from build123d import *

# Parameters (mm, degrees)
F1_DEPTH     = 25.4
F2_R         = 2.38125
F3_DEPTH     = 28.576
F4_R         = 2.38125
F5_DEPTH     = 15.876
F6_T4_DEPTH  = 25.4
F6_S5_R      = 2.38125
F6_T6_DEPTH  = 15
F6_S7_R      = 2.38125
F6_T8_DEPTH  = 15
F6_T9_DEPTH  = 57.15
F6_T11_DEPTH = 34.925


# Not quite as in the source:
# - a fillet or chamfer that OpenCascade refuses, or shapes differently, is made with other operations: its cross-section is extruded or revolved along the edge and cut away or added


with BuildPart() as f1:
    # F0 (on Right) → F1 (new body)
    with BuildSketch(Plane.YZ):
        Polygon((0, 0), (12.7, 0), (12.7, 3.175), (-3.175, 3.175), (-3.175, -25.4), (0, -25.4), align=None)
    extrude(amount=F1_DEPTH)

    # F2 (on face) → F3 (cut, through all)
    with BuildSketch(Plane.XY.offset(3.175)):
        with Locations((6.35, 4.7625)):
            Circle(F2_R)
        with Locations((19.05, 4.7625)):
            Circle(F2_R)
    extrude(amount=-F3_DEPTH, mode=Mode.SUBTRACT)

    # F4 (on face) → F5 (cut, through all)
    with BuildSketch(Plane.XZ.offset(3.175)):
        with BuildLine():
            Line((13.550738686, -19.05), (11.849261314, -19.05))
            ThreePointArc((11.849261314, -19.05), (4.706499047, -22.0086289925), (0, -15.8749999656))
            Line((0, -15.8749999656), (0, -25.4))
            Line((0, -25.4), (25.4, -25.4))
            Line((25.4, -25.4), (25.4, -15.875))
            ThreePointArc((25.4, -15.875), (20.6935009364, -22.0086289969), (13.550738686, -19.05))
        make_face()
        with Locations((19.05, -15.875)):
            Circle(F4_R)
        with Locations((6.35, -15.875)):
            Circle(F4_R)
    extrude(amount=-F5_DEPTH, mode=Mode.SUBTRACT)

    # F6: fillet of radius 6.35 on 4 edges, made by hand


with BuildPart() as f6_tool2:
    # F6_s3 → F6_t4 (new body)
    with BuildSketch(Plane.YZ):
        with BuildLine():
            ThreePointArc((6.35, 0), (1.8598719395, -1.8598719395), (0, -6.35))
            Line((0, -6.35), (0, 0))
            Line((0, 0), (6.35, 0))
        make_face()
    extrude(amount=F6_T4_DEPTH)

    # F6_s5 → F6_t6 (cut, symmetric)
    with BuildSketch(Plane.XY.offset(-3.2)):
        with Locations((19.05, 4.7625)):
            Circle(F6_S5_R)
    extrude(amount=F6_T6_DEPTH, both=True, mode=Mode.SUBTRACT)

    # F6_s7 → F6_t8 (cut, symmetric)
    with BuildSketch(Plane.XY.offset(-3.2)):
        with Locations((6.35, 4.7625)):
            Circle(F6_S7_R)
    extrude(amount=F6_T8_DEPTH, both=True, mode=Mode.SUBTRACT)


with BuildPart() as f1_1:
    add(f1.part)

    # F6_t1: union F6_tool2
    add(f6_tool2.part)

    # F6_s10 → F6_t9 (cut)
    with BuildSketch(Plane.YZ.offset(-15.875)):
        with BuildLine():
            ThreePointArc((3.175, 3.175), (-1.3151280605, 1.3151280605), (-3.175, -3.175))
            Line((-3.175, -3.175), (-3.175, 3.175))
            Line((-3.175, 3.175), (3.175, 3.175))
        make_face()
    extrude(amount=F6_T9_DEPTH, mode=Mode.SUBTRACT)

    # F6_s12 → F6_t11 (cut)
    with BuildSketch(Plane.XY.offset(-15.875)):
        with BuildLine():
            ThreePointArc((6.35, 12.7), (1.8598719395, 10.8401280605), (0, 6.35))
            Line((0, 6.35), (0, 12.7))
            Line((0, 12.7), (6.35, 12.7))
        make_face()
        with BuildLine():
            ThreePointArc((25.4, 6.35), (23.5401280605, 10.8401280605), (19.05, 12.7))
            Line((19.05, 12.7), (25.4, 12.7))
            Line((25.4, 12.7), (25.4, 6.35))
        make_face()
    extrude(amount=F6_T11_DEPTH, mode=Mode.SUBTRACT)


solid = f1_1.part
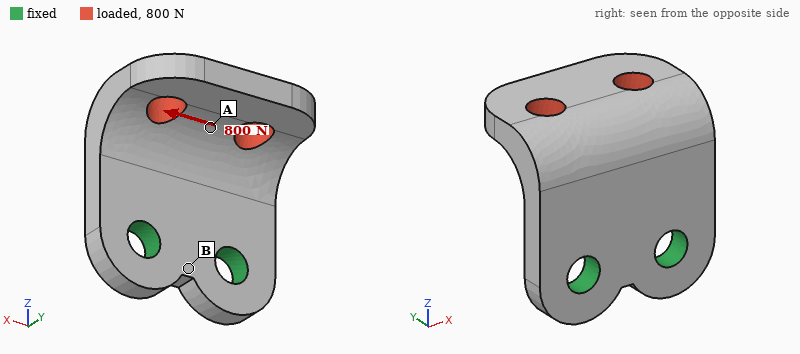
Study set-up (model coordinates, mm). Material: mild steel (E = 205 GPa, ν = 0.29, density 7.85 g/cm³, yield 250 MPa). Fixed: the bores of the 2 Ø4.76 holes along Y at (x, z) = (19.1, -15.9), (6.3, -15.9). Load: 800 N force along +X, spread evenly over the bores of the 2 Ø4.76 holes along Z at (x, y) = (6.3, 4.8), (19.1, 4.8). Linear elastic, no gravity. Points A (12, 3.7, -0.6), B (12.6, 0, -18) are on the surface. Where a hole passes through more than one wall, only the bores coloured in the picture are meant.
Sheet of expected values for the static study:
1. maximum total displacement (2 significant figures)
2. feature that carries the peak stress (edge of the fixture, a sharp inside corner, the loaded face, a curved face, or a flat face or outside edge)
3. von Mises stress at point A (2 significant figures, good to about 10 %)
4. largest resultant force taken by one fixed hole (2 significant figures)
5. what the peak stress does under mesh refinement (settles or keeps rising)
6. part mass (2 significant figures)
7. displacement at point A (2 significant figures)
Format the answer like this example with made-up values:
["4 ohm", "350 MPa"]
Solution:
["26 µm", "edge of the fixture", "50 MPa", "930 N", "keeps rising", "21 g", "10 µm"]
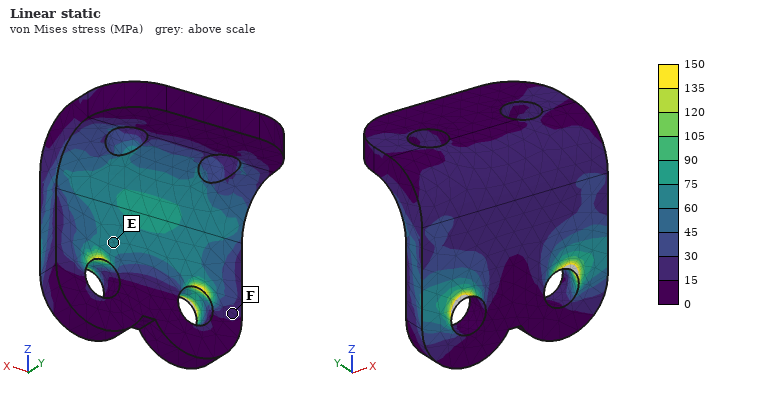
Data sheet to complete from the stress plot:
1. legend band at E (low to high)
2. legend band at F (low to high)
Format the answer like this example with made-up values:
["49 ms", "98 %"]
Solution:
["60 to 75 MPa", "15 to 30 MPa"]
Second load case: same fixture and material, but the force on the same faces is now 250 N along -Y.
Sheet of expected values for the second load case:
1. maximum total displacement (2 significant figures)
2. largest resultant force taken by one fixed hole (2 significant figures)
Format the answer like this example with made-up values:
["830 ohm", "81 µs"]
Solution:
["40 µm", "130 N"]
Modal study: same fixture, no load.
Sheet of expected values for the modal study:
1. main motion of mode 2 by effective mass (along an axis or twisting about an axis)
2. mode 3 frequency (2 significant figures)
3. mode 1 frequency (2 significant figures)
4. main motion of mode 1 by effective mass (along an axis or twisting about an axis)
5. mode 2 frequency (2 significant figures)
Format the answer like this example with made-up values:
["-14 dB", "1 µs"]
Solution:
["along X", "16 kHz", "4400 Hz", "along Y", "8400 Hz"]
